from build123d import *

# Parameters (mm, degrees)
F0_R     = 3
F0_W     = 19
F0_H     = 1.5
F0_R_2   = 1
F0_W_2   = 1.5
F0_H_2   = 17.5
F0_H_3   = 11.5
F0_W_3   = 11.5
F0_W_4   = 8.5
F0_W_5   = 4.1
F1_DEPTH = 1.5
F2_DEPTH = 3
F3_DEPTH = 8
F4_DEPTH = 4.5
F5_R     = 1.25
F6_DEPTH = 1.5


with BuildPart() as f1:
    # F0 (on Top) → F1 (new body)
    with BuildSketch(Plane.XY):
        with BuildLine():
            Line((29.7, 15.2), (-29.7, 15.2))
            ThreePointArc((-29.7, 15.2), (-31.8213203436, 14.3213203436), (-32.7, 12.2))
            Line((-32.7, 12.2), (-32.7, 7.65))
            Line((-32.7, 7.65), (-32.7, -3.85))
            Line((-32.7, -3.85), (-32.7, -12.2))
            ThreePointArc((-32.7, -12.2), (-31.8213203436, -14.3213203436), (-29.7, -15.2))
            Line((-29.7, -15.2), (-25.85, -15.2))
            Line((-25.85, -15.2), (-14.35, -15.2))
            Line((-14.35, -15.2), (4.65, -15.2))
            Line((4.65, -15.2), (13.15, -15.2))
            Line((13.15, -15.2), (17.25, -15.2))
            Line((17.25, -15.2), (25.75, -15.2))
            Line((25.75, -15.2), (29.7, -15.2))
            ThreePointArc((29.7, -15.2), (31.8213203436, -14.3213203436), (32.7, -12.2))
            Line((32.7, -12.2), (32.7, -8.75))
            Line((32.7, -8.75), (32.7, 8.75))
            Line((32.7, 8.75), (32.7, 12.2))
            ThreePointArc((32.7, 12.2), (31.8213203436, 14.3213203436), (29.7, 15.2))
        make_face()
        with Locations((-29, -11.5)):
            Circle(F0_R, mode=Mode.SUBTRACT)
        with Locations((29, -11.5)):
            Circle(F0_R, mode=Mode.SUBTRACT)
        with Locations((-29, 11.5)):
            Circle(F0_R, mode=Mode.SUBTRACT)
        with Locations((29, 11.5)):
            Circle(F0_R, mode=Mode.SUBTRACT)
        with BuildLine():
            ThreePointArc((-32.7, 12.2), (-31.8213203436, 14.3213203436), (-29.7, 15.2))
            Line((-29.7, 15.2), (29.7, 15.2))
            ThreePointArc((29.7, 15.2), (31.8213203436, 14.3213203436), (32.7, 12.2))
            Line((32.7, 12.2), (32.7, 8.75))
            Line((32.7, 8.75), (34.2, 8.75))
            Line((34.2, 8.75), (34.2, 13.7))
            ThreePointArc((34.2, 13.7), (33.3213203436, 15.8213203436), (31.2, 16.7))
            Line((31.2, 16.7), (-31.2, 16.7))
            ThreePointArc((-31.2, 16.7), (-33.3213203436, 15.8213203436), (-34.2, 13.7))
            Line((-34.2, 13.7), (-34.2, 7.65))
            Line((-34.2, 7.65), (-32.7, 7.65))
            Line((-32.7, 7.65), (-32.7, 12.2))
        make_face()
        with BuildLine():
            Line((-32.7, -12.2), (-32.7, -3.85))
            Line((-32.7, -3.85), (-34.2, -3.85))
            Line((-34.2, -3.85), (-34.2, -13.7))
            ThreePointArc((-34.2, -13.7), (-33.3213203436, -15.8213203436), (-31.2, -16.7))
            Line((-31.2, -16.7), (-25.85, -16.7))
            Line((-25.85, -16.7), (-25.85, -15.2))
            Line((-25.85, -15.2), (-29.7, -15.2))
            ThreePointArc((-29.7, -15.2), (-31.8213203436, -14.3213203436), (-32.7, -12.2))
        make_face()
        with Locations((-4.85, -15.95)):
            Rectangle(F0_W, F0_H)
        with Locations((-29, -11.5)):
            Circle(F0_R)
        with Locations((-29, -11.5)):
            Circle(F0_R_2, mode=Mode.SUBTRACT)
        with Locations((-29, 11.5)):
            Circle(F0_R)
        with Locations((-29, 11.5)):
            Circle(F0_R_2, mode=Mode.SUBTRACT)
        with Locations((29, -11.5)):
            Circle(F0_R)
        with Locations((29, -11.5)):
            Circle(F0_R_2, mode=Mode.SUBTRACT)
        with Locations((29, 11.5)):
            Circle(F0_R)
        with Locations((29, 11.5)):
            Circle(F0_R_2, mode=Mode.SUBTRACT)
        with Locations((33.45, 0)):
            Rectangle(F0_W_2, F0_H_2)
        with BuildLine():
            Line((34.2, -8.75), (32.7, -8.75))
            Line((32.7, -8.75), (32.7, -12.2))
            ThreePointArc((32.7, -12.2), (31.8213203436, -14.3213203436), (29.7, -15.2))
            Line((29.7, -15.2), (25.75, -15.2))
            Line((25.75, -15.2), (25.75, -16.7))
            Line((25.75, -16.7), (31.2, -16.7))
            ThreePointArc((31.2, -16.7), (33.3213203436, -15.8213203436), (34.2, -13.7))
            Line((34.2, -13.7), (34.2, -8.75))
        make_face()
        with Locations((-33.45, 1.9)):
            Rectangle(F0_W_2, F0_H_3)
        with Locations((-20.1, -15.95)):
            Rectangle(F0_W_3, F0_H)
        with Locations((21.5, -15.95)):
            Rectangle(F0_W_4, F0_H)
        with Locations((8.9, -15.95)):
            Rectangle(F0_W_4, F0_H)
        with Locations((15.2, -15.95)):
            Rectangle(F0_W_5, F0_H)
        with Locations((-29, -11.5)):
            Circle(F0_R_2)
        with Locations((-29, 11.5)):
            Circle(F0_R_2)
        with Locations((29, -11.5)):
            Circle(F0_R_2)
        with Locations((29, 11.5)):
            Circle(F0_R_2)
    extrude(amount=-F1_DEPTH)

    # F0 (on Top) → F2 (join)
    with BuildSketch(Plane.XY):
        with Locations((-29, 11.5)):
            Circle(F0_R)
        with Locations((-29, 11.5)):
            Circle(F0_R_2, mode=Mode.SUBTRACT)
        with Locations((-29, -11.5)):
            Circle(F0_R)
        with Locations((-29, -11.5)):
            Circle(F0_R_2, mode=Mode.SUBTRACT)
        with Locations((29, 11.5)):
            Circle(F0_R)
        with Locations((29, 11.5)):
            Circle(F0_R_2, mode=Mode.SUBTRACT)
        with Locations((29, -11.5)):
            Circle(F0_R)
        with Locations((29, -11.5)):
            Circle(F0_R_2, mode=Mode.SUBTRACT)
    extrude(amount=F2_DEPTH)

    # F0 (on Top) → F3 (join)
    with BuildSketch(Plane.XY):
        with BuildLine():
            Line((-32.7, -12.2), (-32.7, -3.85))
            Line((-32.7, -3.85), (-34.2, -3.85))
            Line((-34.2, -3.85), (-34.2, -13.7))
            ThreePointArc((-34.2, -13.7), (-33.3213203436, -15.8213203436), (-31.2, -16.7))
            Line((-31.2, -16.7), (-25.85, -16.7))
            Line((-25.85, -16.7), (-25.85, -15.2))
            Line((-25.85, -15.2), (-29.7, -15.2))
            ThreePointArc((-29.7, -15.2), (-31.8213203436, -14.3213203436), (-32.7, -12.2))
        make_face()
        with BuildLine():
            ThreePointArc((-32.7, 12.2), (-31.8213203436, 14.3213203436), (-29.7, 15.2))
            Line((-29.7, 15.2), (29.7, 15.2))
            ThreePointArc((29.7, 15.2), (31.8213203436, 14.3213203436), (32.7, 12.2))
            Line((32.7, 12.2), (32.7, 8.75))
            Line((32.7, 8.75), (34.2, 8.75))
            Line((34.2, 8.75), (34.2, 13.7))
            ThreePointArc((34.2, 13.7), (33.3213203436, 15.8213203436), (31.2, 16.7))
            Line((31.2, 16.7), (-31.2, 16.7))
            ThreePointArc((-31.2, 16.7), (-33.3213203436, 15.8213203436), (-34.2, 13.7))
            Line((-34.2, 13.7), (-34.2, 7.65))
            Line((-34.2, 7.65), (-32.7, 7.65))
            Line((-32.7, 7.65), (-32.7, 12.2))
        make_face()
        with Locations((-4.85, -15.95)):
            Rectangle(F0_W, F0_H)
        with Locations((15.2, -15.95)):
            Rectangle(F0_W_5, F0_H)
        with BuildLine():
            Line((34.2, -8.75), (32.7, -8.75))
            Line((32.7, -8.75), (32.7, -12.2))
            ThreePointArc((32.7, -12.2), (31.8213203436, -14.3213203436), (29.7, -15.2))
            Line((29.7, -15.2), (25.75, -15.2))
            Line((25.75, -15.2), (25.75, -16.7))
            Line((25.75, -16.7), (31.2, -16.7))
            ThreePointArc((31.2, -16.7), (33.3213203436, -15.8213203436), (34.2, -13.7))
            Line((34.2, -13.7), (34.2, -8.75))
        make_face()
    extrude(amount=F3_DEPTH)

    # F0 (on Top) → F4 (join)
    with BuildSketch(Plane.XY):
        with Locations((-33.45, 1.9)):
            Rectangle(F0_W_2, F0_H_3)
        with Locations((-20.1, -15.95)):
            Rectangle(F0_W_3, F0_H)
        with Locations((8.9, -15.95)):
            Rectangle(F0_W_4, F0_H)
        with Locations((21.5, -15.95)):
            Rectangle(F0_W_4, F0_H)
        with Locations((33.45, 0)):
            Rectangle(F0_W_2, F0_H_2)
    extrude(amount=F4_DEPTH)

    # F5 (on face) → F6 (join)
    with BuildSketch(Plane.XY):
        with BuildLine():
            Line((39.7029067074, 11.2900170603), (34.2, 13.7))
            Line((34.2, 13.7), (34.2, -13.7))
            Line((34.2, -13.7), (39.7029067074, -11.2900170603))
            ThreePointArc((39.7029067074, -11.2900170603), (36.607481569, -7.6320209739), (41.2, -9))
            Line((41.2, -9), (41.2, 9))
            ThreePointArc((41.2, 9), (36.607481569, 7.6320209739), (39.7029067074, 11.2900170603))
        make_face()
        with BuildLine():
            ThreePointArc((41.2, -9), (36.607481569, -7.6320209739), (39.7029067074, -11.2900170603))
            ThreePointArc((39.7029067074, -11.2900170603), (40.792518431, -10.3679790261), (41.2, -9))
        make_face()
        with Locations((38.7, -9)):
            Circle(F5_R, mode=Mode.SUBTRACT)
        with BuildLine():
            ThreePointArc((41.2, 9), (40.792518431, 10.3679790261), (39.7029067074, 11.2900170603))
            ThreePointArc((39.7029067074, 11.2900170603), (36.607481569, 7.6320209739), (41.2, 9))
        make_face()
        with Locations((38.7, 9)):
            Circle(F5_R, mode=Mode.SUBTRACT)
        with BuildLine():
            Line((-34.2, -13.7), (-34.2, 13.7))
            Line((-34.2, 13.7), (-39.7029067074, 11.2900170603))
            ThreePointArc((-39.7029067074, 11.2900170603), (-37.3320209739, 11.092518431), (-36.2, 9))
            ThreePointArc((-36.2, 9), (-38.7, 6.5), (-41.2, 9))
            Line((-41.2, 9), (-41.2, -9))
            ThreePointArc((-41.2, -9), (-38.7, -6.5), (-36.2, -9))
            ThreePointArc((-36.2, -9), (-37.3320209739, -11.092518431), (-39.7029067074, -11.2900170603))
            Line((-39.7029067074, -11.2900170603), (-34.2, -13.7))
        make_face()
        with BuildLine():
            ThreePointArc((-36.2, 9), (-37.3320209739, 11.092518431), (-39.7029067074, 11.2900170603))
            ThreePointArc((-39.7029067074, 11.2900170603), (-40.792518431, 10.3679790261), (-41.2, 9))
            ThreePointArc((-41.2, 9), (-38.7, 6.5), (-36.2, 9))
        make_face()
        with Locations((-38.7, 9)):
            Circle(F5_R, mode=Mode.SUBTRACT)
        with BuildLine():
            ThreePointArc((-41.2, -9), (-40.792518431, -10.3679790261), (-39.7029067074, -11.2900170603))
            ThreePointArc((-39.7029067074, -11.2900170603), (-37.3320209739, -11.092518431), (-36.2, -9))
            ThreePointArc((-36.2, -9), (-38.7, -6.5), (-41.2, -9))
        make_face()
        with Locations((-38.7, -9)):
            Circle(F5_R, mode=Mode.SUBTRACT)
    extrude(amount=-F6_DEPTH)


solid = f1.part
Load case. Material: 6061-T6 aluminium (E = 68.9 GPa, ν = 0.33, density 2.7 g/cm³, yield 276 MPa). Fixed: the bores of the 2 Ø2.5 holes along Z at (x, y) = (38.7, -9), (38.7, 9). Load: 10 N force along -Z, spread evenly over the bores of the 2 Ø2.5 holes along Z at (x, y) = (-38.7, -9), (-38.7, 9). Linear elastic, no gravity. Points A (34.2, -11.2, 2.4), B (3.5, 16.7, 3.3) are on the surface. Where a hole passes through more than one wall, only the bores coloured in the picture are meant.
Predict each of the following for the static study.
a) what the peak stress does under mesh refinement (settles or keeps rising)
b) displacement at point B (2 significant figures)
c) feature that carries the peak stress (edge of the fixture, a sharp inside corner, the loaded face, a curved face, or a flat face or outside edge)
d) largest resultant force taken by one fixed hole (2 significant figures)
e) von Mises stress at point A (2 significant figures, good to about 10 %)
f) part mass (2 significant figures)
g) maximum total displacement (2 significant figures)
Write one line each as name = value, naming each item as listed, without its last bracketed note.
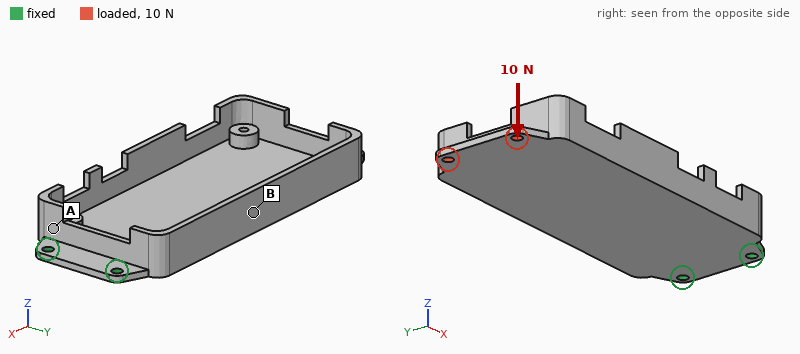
what the peak stress does under mesh refinement = keeps rising
displacement at point B = 0.34 mm
feature that carries the peak stress = edge of the fixture
largest resultant force taken by one fixed hole = 25 N
von Mises stress at point A = 17 MPa
part mass = 17 g
maximum total displacement = 0.84 mm
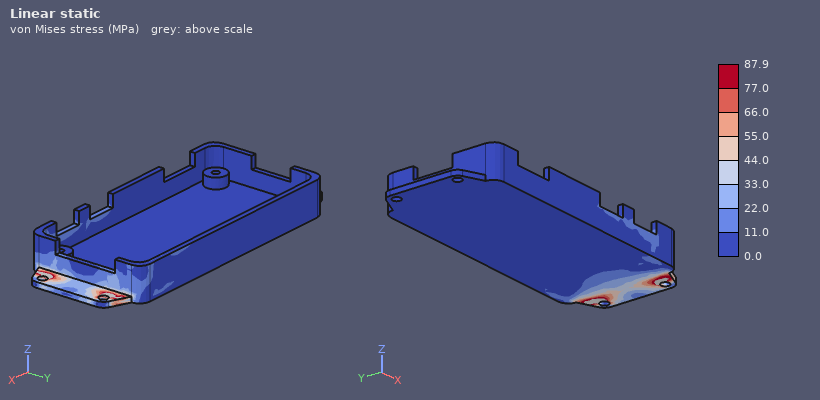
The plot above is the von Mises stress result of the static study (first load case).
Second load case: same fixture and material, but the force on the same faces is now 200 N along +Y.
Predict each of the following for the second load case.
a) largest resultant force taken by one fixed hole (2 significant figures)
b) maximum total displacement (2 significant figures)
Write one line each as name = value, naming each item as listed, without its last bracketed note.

largest resultant force taken by one fixed hole = 820 N
maximum total displacement = 0.15 mm
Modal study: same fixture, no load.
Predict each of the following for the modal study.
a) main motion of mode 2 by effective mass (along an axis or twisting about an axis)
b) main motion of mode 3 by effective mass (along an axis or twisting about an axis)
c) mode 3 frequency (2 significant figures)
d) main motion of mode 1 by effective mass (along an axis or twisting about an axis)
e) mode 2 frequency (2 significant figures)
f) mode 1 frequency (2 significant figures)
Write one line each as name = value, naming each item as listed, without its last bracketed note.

main motion of mode 2 by effective mass = twisting about X
main motion of mode 3 by effective mass = along Y
mode 3 frequency = 2500 Hz
main motion of mode 1 by effective mass = along Z
mode 2 frequency = 890 Hz
mode 1 frequency = 240 Hz
